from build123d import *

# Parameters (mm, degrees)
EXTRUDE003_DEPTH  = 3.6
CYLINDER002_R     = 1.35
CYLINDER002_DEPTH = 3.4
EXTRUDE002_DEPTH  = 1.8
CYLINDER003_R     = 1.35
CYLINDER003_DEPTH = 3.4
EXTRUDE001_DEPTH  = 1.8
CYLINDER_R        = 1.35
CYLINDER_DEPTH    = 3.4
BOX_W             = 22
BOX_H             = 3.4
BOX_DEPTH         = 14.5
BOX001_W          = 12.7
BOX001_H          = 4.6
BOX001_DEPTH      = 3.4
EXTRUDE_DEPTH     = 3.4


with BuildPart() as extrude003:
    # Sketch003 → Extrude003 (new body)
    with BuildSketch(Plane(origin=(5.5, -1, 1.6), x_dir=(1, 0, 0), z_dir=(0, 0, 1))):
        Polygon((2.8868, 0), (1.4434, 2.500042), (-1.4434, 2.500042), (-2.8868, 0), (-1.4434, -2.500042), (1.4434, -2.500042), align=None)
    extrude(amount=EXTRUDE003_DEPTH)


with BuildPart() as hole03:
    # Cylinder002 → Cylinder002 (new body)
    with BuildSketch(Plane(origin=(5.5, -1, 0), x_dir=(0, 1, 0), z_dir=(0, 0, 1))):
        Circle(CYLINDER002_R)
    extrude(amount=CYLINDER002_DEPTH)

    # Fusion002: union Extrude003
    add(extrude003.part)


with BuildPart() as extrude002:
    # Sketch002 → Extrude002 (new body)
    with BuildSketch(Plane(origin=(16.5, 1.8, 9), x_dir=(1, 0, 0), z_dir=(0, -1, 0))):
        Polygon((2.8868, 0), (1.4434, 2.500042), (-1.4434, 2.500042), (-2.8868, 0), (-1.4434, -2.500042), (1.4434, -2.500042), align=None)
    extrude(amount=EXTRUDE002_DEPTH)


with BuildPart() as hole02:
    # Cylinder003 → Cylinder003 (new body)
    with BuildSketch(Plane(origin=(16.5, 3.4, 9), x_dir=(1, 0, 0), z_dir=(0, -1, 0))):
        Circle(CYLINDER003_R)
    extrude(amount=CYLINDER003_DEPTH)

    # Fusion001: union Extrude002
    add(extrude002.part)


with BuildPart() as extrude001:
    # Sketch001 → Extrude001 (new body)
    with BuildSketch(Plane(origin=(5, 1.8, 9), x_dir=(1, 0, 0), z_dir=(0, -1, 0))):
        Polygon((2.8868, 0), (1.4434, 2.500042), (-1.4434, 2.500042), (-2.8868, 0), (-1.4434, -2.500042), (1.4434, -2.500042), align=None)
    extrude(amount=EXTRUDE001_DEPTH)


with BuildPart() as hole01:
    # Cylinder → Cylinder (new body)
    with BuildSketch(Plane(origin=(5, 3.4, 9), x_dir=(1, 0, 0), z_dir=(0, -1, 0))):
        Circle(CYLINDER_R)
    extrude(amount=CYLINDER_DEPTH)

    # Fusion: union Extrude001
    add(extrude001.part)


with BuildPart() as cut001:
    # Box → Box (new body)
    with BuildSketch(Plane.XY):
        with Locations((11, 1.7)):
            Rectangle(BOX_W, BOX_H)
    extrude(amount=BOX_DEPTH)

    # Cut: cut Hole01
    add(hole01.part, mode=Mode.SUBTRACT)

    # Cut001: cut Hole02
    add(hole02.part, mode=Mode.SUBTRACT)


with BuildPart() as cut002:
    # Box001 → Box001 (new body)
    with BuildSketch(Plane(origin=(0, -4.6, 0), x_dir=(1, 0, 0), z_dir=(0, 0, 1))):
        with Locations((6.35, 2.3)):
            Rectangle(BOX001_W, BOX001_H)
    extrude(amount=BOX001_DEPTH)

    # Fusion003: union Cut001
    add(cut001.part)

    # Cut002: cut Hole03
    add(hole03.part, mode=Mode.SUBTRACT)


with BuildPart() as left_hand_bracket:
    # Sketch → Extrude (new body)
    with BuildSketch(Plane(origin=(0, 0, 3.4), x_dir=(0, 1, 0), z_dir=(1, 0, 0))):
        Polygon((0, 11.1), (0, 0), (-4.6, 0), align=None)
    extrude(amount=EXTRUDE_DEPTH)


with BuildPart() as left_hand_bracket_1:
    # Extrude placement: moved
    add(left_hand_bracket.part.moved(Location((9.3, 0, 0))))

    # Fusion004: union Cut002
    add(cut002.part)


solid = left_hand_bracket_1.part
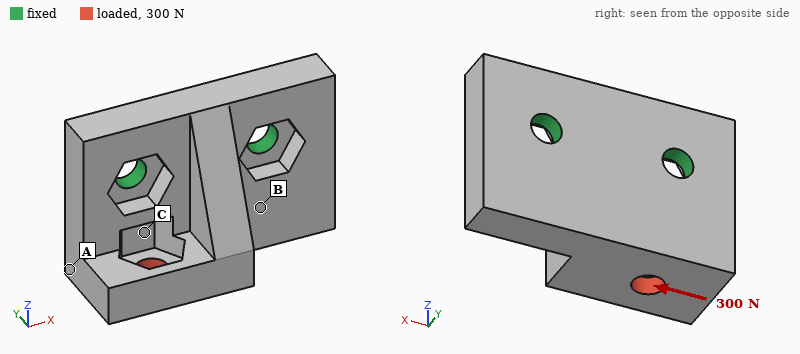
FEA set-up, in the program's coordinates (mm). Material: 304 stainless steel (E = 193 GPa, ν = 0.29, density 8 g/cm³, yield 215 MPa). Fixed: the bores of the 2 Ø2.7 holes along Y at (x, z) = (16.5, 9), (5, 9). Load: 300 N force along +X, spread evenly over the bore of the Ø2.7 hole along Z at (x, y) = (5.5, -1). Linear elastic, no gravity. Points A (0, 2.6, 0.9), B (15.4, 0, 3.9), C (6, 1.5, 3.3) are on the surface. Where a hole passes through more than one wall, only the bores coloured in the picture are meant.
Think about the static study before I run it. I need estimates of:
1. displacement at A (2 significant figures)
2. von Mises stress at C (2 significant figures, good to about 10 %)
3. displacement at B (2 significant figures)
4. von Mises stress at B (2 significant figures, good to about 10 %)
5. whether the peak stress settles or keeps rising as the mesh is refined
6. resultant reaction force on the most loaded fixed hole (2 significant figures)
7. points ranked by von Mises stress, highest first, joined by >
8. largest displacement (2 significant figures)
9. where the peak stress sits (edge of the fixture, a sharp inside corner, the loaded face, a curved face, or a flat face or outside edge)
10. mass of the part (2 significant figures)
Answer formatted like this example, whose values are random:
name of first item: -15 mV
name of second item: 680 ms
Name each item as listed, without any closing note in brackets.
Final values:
displacement at A: 2.3 µm
von Mises stress at C: 21 MPa
displacement at B: 0.77 µm
von Mises stress at B: 13 MPa
whether the peak stress settles or keeps rising as the mesh is refined: keeps rising
resultant reaction force on the most loaded fixed hole: 270 N
points ranked by von Mises stress, highest first, joined by >: C > B > A
largest displacement: 3.2 µm
where the peak stress sits: edge of the fixture
mass of the part: 9.7 g
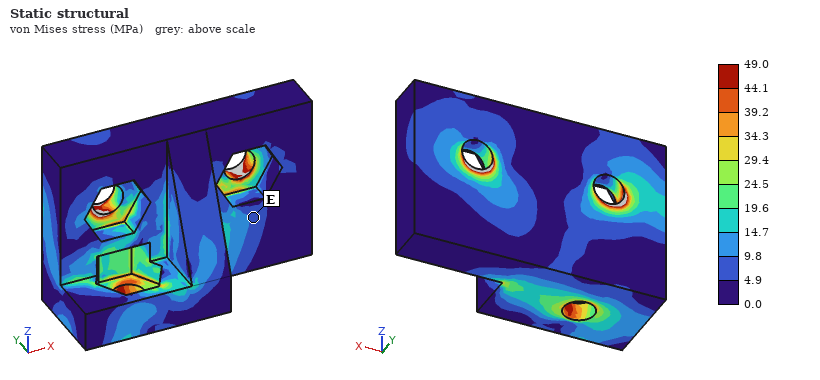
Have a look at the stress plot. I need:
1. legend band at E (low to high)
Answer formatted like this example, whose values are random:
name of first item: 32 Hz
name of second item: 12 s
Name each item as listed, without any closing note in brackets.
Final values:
legend band at E: 4.9 to 9.8 MPa
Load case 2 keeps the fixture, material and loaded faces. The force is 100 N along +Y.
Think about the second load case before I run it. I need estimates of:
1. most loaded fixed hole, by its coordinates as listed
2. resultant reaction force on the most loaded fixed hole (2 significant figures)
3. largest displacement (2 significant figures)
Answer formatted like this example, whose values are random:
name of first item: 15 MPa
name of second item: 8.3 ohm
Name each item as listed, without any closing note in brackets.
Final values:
most loaded fixed hole, by its coordinates as listed: (5, 9)
resultant reaction force on the most loaded fixed hole: 94 N
largest displacement: 6.7 µm
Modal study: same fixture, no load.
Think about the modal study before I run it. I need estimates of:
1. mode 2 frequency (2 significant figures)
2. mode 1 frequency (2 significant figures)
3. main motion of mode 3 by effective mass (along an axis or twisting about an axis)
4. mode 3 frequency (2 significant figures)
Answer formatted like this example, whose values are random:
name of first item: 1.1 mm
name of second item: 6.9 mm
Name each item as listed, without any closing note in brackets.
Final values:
mode 2 frequency: 25 kHz
mode 1 frequency: 13 kHz
main motion of mode 3 by effective mass: along X
mode 3 frequency: 37 kHz
